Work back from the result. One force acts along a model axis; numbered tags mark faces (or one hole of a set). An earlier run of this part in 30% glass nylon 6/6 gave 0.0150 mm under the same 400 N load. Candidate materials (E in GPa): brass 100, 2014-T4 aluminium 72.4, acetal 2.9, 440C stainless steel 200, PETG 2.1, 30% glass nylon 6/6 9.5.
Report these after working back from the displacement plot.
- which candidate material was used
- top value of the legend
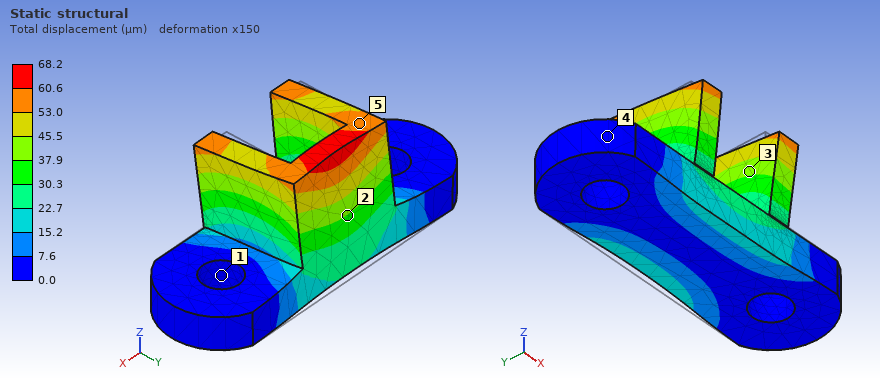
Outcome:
PETG
68.2 µm
